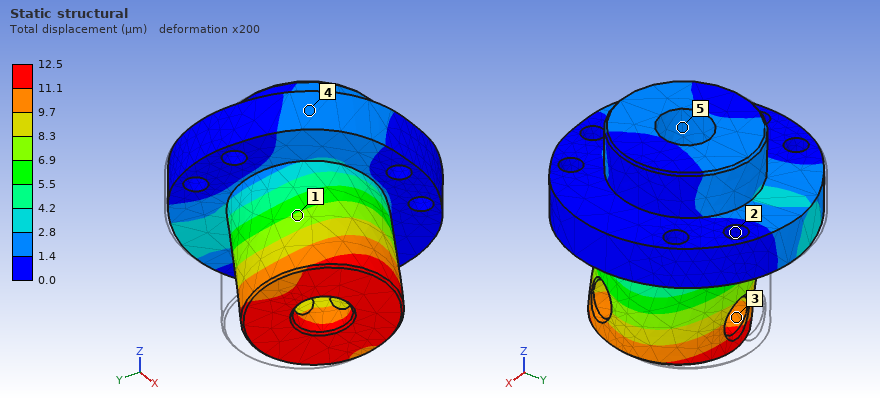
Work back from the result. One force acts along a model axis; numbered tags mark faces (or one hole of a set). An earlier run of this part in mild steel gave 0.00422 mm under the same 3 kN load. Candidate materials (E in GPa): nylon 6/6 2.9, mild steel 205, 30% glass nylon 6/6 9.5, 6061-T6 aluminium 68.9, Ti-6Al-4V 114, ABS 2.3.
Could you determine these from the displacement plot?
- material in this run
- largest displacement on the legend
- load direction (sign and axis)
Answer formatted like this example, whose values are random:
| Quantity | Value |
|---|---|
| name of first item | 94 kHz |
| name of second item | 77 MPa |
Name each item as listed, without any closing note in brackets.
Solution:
| Quantity | Value |
|---|---|
| material in this run | 6061-T6 aluminium |
| largest displacement on the legend | 12.5 µm |
| load direction | -Y |
